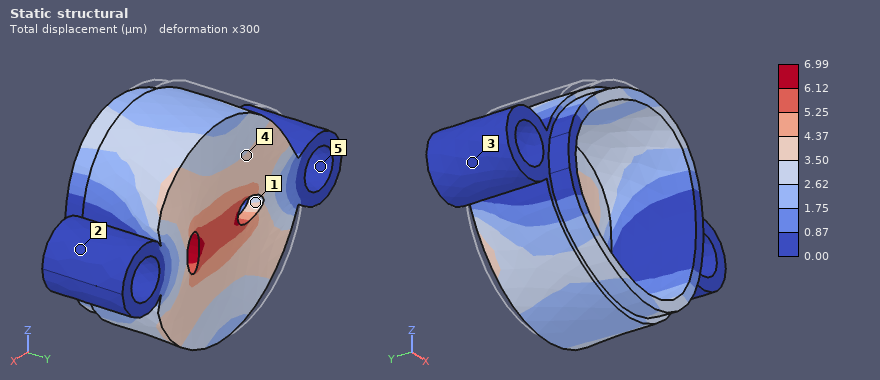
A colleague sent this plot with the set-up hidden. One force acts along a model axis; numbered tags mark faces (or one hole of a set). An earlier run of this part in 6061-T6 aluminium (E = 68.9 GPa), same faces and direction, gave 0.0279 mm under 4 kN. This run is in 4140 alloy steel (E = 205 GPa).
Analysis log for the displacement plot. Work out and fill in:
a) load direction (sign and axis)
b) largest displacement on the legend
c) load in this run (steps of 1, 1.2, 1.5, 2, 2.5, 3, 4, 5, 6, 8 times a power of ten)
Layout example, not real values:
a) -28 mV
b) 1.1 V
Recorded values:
a) +X
b) 6.99 µm
c) 3 kN
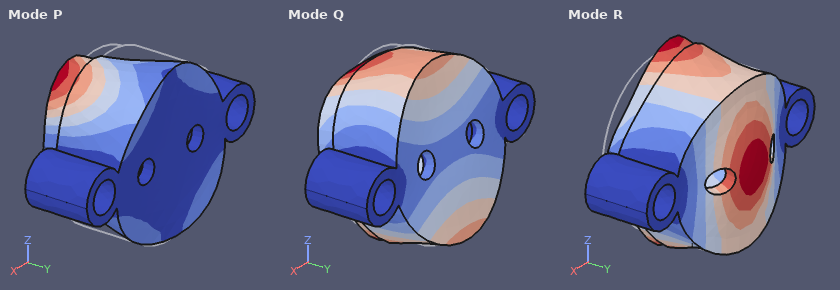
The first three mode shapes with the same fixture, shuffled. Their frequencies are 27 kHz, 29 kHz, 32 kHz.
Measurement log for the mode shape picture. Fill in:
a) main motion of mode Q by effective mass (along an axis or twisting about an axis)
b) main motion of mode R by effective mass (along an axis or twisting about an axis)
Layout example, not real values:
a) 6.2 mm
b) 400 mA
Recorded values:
a) twisting about X
b) along Y
